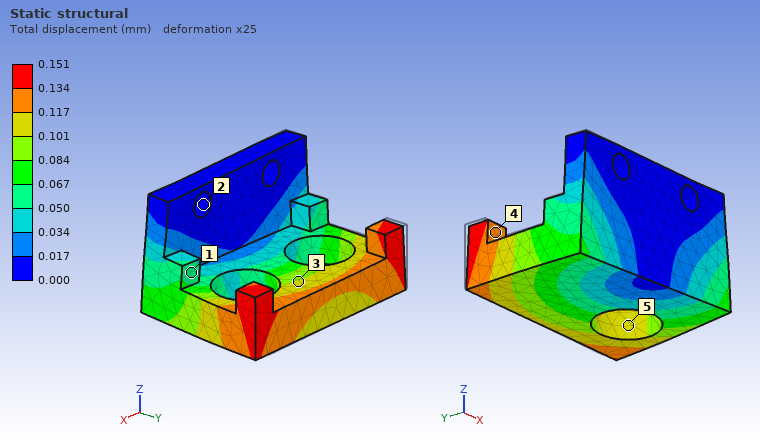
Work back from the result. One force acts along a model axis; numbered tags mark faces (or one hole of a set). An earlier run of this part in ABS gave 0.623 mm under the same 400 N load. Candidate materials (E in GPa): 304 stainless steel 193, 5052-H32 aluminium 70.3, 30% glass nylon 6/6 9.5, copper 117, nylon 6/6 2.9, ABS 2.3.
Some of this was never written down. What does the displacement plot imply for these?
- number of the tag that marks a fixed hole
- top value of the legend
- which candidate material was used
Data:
2
0.151 mm
30% glass nylon 6/6
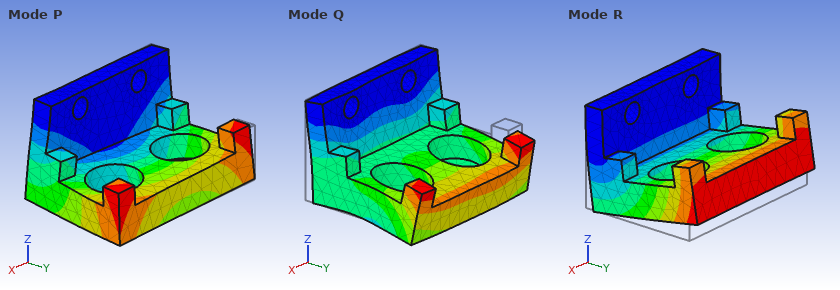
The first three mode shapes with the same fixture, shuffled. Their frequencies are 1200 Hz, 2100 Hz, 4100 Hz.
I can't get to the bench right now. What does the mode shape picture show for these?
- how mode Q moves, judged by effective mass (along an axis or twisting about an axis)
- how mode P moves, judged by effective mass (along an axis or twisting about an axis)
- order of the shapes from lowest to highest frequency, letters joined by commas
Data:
along Y
along X
R, P, Q
